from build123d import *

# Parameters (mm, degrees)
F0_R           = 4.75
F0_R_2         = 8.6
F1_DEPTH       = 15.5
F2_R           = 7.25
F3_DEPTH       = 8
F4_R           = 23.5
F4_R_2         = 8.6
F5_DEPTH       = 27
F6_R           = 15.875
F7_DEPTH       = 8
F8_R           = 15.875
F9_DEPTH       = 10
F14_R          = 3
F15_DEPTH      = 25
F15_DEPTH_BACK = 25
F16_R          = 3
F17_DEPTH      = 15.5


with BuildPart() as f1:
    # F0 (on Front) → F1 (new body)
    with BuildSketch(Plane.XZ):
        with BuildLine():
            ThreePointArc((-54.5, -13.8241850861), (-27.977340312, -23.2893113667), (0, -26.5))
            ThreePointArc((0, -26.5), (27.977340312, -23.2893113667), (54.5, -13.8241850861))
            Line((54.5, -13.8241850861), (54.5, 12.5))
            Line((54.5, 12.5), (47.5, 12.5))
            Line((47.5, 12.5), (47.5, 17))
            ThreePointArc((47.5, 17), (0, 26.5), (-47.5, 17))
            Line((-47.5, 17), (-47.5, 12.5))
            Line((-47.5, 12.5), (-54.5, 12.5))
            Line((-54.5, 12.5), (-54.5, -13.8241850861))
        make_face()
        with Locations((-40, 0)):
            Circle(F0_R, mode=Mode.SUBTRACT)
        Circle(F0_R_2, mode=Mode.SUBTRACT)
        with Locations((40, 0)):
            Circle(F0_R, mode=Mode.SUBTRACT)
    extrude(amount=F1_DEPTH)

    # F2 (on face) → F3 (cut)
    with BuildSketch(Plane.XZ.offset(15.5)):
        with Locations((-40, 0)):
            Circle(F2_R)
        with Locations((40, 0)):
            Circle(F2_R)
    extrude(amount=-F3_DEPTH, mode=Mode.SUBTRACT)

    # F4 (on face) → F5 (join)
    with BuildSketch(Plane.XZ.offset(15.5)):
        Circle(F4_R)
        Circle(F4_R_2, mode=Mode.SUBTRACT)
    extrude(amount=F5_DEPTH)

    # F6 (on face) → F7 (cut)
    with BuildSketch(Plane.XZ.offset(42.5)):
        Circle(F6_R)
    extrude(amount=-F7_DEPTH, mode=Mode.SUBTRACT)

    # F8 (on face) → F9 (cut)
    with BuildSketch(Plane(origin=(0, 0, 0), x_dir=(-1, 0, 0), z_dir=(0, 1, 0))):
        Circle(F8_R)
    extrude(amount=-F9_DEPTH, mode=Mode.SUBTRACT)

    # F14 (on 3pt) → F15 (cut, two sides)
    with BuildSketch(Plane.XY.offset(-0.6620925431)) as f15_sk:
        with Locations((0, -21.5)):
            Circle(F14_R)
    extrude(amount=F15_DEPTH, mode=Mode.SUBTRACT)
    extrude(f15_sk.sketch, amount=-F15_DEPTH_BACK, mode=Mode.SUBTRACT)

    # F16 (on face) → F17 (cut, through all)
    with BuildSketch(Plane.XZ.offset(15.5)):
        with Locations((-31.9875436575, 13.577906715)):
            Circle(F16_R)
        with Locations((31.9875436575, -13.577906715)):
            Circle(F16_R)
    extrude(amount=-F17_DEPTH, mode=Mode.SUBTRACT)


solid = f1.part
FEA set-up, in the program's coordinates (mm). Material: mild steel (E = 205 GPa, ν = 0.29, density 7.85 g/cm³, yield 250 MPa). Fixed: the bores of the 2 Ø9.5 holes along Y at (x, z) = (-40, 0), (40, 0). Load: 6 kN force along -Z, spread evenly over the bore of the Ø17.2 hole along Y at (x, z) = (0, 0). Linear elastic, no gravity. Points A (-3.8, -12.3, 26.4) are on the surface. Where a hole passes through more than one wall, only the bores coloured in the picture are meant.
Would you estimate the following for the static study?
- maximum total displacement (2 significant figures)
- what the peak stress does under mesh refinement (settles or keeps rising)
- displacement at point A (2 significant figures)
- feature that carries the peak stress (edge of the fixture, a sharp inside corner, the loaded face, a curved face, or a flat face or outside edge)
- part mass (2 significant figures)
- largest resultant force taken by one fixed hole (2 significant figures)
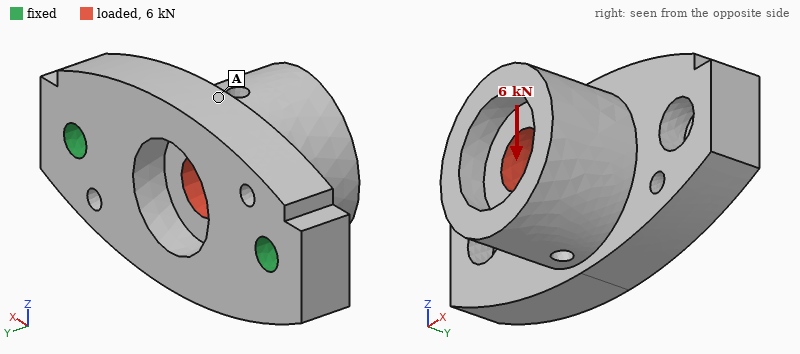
36 µm
keeps rising
22 µm
edge of the fixture
760 g
3.0 kN
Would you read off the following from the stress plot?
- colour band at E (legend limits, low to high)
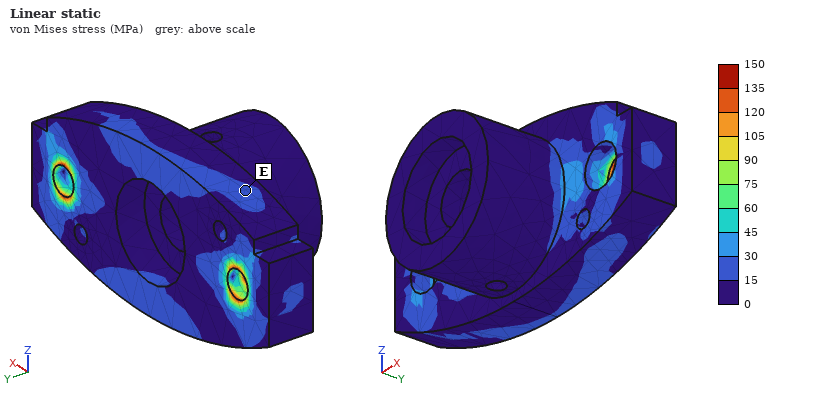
15 to 30 MPa
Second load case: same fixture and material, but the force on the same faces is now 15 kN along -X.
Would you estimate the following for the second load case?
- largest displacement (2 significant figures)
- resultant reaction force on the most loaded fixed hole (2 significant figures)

8.3 µm
8.3 kN
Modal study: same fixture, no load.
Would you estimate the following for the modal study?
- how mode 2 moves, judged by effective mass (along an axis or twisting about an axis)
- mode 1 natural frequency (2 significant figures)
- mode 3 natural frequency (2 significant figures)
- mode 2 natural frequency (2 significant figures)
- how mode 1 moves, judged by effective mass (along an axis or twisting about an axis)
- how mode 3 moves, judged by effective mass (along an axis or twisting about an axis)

along Y
3300 Hz
11 kHz
7100 Hz
along Z
along X
